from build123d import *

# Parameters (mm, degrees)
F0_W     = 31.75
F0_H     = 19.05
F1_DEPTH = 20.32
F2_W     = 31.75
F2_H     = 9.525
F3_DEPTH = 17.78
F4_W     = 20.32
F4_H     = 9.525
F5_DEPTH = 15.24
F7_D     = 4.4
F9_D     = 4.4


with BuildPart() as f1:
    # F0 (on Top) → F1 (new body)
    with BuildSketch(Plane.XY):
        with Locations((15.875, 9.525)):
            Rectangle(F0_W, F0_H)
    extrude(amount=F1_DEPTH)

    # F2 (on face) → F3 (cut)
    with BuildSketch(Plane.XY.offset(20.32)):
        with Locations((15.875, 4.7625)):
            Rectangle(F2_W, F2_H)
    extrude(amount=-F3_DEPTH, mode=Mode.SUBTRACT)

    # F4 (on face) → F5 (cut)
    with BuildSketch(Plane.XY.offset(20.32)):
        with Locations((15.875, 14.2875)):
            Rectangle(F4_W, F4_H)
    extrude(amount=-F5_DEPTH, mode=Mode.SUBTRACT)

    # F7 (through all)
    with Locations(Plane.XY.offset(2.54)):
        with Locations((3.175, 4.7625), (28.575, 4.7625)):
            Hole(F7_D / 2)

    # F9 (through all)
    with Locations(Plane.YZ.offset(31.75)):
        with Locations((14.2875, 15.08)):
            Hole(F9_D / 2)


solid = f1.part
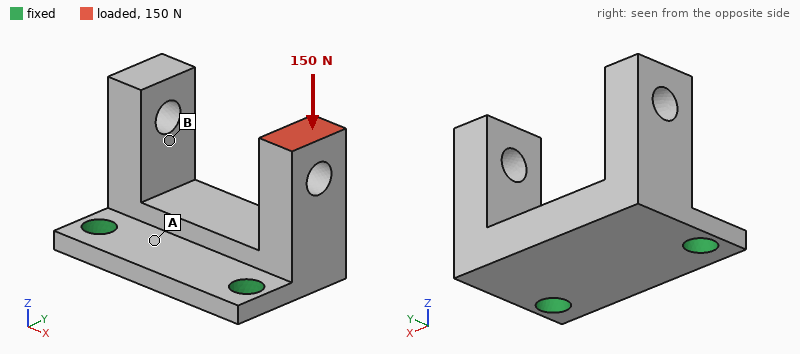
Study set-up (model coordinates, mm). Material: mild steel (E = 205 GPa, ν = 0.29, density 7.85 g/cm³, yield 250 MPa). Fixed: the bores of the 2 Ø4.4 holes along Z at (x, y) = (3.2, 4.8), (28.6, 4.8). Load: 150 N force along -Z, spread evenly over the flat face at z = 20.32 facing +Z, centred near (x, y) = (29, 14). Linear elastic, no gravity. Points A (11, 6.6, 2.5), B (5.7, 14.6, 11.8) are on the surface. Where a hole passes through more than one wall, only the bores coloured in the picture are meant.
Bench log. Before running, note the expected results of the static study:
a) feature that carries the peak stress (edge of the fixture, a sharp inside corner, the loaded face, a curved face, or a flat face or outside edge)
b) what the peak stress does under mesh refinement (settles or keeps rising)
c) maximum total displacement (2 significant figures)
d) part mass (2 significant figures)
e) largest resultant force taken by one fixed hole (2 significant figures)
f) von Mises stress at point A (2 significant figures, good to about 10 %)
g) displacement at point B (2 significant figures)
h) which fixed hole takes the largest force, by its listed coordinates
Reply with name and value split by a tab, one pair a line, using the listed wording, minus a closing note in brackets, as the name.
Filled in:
feature that carries the peak stress	edge of the fixture
what the peak stress does under mesh refinement	keeps rising
maximum total displacement	17 µm
part mass	29 g
largest resultant force taken by one fixed hole	150 N
von Mises stress at point A	12 MPa
displacement at point B	5.7 µm
which fixed hole takes the largest force, by its listed coordinates	(28.6, 4.8)
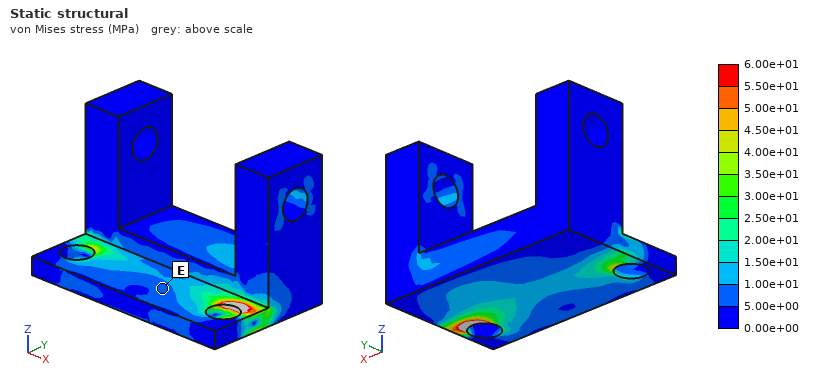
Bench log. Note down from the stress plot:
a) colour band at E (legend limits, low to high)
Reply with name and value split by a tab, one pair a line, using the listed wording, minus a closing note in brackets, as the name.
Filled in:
colour band at E	5.00e+00 to 1.00e+01 MPa
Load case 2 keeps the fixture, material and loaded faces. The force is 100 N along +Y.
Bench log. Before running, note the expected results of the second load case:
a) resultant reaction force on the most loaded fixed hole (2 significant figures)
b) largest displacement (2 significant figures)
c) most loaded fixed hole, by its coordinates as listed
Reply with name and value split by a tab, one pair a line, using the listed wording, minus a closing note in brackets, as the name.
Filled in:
resultant reaction force on the most loaded fixed hole	100 N
largest displacement	39 µm
most loaded fixed hole, by its coordinates as listed	(28.6, 4.8)
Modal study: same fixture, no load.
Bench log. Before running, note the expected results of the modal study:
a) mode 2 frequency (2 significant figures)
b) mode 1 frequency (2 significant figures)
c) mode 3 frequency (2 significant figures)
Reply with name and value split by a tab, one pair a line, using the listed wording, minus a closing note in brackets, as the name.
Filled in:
mode 2 frequency	6600 Hz
mode 1 frequency	3600 Hz
mode 3 frequency	8600 Hz
